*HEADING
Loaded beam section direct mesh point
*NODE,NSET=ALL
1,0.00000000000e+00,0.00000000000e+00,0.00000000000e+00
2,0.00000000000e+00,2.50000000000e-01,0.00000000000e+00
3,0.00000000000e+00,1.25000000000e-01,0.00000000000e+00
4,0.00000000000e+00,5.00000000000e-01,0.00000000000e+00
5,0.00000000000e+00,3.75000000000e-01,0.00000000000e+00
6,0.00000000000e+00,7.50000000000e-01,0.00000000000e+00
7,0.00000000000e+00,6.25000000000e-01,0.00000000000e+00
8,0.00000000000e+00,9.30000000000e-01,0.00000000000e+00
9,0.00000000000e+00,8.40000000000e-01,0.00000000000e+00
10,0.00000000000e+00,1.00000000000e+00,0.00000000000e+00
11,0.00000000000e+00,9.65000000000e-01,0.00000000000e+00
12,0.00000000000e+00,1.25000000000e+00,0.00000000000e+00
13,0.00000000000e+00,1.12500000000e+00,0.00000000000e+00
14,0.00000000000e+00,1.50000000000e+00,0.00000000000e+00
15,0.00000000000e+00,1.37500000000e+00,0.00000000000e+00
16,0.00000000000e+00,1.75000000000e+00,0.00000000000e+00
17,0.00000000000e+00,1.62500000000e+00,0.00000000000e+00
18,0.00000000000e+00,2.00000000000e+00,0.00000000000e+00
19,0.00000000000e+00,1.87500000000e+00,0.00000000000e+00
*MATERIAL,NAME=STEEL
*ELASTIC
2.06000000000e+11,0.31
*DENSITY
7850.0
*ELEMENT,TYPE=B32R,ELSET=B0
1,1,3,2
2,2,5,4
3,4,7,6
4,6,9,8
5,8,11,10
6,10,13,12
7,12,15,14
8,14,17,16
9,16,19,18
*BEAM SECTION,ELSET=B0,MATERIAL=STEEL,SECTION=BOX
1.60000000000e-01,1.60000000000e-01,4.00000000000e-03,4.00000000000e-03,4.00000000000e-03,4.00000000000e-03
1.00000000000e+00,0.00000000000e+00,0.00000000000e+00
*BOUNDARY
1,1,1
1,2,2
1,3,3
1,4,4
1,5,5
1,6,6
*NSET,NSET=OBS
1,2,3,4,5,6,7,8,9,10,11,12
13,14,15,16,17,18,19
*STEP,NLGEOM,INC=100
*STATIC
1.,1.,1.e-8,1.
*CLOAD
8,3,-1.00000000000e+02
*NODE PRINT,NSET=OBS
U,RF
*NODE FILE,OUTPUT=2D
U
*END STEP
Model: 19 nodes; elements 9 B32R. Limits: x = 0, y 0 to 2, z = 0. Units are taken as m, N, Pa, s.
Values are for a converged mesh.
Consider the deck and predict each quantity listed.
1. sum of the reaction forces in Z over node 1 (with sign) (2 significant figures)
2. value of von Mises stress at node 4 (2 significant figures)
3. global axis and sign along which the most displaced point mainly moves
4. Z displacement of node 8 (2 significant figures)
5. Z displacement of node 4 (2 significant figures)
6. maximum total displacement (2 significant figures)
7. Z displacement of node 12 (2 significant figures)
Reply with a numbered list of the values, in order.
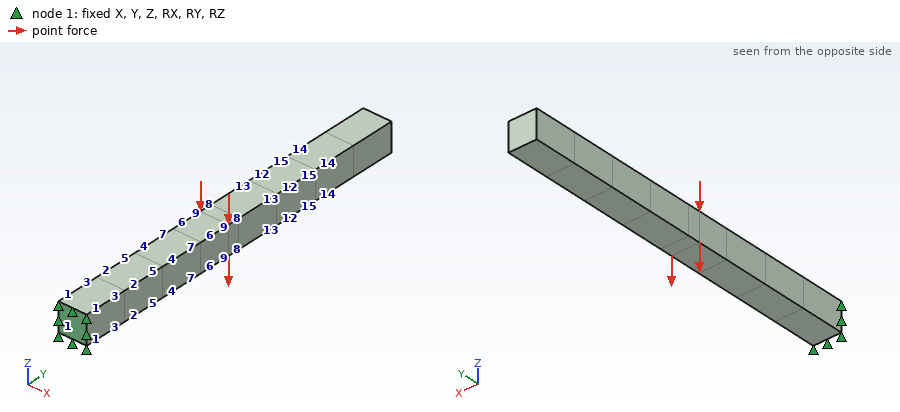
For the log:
1. 100 N
2. 3.5e+05 Pa
3. -Z
4. -1.3e-05 m
5. -4.7e-06 m
6. 3.5e-05 m
7. -2.0e-05 m
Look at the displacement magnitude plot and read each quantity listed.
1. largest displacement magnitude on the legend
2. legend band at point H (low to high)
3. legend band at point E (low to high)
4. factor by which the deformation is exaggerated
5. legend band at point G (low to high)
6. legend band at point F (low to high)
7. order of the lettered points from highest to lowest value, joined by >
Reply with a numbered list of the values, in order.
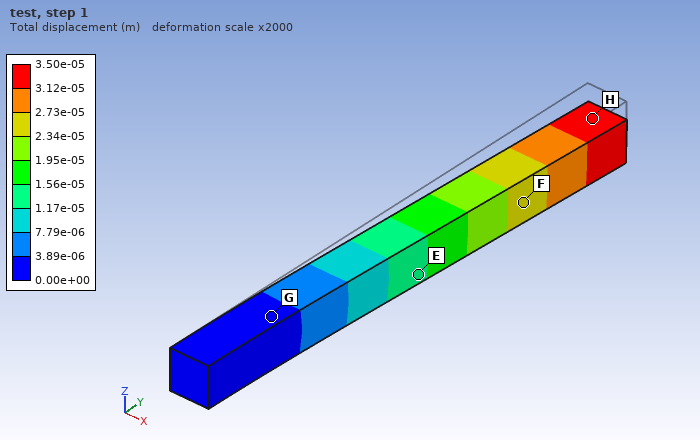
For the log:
1. 3.50e-05 m
2. 3.12e-05 to 3.50e-05 m
3. 1.17e-05 to 1.56e-05 m
4. 2000
5. 0.00e+00 to 3.89e-06 m
6. 2.34e-05 to 2.73e-05 m
7. H > F > E > G
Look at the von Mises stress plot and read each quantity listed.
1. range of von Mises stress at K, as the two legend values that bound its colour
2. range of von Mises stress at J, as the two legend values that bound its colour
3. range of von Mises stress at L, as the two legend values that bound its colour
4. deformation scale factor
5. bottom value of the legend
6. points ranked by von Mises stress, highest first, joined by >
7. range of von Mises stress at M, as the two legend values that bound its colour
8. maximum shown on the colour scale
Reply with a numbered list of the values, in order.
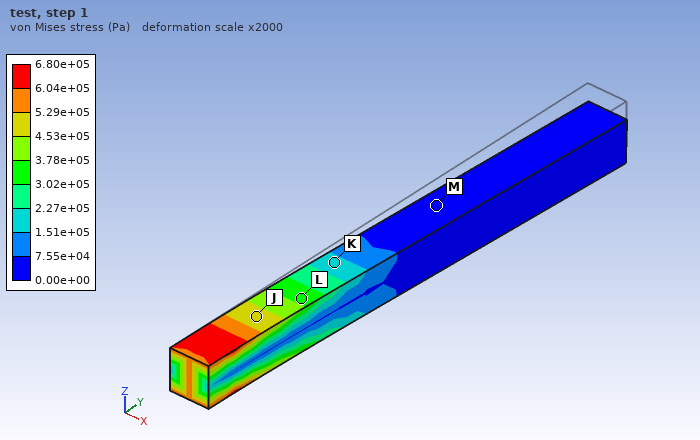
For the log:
1. 1.51e+05 to 2.27e+05 Pa
2. 4.53e+05 to 5.29e+05 Pa
3. 3.02e+05 to 3.78e+05 Pa
4. 2000
5. 0.00e+00 Pa
6. J > L > K > M
7. 0.00e+00 to 7.55e+04 Pa
8. 6.80e+05 Pa
